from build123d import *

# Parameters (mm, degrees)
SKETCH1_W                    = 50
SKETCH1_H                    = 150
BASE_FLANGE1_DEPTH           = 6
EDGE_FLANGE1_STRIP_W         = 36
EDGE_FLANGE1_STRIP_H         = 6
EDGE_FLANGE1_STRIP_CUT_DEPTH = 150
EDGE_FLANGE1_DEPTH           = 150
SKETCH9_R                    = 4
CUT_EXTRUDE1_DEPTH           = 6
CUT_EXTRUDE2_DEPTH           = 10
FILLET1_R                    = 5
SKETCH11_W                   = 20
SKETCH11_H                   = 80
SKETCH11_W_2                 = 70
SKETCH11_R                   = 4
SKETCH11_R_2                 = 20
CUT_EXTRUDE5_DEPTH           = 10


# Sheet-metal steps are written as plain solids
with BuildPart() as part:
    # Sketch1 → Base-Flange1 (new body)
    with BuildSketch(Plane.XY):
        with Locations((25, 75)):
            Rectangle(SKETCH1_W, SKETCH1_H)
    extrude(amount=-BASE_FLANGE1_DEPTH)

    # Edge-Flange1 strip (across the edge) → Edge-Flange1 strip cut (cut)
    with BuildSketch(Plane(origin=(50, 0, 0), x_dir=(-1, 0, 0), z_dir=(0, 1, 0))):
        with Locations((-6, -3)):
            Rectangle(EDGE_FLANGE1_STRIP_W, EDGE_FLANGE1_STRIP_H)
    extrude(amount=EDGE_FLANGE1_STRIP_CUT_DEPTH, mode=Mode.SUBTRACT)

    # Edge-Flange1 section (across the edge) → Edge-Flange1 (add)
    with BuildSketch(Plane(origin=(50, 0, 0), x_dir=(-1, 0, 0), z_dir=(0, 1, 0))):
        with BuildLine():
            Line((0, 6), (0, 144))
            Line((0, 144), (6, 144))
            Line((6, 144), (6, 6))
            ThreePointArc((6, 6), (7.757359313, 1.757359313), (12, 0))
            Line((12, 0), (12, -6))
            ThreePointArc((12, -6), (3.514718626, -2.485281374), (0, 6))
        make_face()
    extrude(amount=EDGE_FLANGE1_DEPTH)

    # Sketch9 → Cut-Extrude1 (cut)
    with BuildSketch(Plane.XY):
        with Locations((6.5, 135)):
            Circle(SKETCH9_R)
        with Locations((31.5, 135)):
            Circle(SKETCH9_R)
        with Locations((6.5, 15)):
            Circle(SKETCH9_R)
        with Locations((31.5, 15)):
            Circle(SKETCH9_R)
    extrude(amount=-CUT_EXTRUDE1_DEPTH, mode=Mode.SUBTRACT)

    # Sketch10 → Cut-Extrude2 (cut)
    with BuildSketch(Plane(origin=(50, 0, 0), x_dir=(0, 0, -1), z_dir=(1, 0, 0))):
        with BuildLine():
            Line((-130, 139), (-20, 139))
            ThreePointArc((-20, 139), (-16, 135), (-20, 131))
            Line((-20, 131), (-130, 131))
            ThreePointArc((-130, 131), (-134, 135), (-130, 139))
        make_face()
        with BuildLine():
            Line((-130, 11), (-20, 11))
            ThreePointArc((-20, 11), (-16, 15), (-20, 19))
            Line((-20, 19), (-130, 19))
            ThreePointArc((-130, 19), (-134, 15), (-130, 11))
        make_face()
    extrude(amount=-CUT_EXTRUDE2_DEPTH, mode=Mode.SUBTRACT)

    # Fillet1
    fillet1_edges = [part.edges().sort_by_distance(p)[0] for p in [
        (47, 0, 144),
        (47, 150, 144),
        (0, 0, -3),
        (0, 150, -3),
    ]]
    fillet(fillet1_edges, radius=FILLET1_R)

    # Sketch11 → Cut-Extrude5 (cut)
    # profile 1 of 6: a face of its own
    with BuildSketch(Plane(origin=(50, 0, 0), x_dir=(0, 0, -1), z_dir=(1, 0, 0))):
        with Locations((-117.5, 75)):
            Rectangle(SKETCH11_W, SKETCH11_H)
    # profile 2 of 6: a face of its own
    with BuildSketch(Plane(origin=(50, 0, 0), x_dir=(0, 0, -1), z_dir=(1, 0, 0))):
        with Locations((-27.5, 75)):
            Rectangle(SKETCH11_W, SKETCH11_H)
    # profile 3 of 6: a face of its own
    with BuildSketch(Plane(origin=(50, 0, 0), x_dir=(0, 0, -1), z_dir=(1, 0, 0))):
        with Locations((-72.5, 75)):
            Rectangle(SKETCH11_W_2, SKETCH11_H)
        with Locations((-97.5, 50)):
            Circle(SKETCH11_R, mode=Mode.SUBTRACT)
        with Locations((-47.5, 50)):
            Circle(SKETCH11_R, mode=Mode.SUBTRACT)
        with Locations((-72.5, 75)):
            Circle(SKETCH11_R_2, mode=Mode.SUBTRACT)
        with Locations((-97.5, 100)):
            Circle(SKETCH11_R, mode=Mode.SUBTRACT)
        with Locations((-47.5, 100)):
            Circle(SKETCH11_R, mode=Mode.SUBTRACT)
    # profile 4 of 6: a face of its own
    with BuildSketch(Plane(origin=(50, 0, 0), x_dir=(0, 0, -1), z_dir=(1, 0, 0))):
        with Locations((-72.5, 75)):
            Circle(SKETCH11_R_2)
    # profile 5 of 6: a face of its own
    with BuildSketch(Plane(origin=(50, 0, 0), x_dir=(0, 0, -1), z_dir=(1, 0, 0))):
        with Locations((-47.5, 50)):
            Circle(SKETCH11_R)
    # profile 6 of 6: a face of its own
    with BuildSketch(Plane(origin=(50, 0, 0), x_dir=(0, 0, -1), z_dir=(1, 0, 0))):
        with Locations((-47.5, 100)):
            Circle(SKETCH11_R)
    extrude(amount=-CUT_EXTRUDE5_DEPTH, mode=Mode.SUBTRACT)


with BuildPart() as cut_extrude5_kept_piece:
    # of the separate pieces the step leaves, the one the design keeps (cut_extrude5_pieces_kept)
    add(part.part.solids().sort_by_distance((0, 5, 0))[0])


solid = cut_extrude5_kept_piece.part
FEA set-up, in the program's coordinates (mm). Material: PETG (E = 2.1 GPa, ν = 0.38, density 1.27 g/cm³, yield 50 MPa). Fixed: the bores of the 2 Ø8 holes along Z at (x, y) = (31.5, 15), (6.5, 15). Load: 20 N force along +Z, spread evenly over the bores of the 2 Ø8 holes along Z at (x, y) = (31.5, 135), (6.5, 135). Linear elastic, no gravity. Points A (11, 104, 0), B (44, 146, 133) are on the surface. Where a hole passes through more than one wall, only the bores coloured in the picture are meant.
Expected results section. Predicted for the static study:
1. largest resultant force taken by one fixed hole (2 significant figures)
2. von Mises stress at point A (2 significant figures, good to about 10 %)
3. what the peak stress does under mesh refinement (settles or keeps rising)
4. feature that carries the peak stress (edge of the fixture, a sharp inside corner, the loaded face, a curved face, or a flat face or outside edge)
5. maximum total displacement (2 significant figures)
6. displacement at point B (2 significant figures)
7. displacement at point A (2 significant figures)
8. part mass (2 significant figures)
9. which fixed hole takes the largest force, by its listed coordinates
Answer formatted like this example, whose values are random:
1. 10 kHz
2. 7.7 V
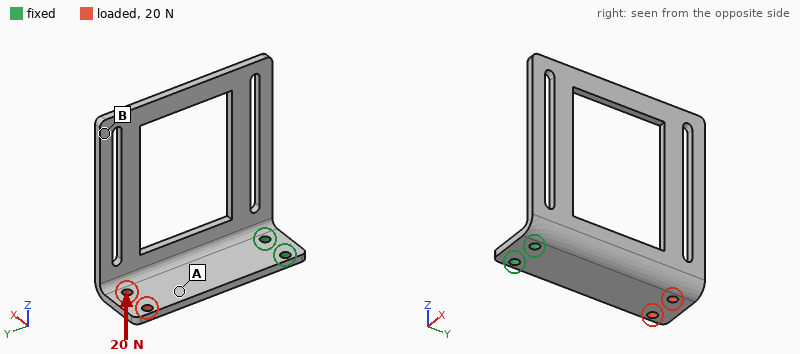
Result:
1. 16 N
2. 1.0 MPa
3. keeps rising
4. edge of the fixture
5. 2.2 mm
6. 2.1 mm
7. 1.1 mm
8. 130 g
9. (31.5, 15)
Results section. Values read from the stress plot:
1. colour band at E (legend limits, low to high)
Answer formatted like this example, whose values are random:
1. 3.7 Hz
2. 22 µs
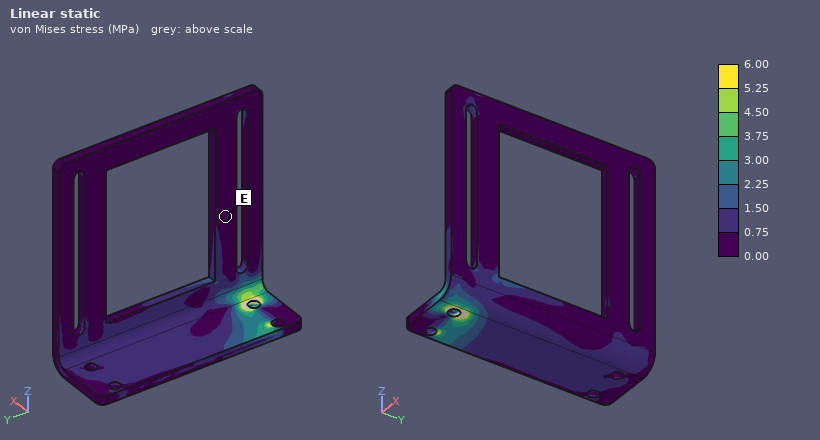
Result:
1. 0.00 to 0.75 MPa
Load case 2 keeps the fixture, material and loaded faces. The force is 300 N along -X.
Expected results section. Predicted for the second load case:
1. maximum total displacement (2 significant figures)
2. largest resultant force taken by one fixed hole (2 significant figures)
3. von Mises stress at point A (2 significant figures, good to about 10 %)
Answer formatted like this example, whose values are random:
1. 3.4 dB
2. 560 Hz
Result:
1. 2.4 mm
2. 1.2 kN
3. 2.7 MPa
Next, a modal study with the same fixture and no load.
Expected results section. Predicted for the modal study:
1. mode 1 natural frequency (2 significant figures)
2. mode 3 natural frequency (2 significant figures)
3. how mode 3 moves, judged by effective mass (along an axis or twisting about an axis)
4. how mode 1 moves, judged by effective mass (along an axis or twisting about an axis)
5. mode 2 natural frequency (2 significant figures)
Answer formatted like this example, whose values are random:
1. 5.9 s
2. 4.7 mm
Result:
1. 38 Hz
2. 92 Hz
3. twisting about Z
4. along X
5. 60 Hz
